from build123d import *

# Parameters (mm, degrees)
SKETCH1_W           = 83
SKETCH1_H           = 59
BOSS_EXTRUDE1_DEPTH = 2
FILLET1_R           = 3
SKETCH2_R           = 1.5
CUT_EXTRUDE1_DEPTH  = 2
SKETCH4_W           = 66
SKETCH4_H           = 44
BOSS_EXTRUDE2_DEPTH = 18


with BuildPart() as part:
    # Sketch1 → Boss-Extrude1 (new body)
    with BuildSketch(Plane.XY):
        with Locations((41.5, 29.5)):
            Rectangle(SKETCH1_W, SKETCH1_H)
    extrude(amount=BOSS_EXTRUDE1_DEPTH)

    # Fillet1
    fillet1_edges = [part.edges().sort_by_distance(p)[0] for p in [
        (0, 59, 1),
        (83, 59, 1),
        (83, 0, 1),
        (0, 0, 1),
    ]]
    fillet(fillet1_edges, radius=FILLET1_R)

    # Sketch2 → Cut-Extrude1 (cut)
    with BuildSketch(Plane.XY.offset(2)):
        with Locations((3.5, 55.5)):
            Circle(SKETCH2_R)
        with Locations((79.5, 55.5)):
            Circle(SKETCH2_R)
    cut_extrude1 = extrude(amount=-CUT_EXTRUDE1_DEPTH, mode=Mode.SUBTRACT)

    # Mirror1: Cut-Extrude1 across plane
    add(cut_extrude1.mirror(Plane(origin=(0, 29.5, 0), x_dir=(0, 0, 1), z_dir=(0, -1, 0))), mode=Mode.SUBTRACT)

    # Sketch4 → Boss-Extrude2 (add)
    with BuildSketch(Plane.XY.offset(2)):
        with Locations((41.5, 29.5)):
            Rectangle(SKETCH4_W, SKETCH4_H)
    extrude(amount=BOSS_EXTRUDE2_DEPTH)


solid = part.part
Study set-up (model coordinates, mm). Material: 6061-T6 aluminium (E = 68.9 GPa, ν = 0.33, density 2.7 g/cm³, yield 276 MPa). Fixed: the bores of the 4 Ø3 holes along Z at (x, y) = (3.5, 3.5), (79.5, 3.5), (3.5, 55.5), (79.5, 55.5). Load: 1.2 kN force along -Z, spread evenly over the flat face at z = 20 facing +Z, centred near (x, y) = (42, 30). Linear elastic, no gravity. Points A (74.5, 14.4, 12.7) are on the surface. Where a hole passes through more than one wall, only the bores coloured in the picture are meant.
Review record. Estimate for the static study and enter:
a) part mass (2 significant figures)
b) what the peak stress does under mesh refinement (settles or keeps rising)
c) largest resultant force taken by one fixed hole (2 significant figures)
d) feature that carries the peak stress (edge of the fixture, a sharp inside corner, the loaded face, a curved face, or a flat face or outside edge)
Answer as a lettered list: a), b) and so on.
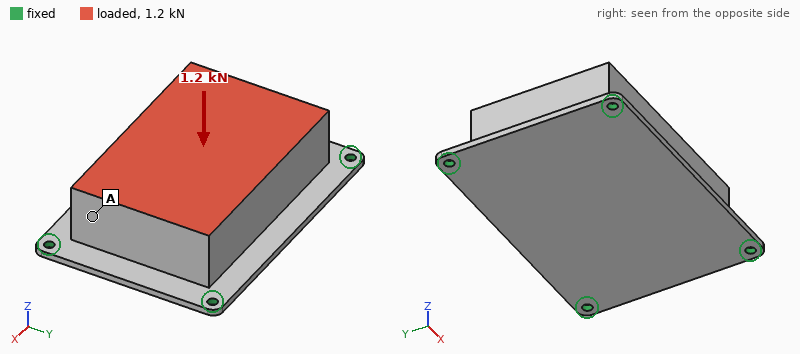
a) 170 g
b) keeps rising
c) 350 N
d) edge of the fixture
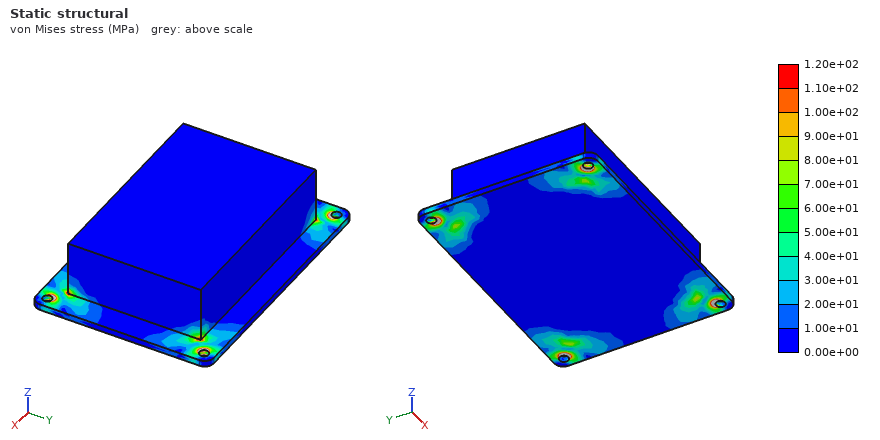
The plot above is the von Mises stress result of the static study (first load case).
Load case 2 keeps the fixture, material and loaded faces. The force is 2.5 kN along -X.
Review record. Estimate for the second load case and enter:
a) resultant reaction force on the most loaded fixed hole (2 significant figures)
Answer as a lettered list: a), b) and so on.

a) 770 N
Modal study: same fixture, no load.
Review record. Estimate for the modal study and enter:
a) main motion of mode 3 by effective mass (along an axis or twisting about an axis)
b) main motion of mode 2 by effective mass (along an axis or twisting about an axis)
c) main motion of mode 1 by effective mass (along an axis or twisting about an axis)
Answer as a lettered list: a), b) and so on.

a) along X
b) along Y
c) along Z
